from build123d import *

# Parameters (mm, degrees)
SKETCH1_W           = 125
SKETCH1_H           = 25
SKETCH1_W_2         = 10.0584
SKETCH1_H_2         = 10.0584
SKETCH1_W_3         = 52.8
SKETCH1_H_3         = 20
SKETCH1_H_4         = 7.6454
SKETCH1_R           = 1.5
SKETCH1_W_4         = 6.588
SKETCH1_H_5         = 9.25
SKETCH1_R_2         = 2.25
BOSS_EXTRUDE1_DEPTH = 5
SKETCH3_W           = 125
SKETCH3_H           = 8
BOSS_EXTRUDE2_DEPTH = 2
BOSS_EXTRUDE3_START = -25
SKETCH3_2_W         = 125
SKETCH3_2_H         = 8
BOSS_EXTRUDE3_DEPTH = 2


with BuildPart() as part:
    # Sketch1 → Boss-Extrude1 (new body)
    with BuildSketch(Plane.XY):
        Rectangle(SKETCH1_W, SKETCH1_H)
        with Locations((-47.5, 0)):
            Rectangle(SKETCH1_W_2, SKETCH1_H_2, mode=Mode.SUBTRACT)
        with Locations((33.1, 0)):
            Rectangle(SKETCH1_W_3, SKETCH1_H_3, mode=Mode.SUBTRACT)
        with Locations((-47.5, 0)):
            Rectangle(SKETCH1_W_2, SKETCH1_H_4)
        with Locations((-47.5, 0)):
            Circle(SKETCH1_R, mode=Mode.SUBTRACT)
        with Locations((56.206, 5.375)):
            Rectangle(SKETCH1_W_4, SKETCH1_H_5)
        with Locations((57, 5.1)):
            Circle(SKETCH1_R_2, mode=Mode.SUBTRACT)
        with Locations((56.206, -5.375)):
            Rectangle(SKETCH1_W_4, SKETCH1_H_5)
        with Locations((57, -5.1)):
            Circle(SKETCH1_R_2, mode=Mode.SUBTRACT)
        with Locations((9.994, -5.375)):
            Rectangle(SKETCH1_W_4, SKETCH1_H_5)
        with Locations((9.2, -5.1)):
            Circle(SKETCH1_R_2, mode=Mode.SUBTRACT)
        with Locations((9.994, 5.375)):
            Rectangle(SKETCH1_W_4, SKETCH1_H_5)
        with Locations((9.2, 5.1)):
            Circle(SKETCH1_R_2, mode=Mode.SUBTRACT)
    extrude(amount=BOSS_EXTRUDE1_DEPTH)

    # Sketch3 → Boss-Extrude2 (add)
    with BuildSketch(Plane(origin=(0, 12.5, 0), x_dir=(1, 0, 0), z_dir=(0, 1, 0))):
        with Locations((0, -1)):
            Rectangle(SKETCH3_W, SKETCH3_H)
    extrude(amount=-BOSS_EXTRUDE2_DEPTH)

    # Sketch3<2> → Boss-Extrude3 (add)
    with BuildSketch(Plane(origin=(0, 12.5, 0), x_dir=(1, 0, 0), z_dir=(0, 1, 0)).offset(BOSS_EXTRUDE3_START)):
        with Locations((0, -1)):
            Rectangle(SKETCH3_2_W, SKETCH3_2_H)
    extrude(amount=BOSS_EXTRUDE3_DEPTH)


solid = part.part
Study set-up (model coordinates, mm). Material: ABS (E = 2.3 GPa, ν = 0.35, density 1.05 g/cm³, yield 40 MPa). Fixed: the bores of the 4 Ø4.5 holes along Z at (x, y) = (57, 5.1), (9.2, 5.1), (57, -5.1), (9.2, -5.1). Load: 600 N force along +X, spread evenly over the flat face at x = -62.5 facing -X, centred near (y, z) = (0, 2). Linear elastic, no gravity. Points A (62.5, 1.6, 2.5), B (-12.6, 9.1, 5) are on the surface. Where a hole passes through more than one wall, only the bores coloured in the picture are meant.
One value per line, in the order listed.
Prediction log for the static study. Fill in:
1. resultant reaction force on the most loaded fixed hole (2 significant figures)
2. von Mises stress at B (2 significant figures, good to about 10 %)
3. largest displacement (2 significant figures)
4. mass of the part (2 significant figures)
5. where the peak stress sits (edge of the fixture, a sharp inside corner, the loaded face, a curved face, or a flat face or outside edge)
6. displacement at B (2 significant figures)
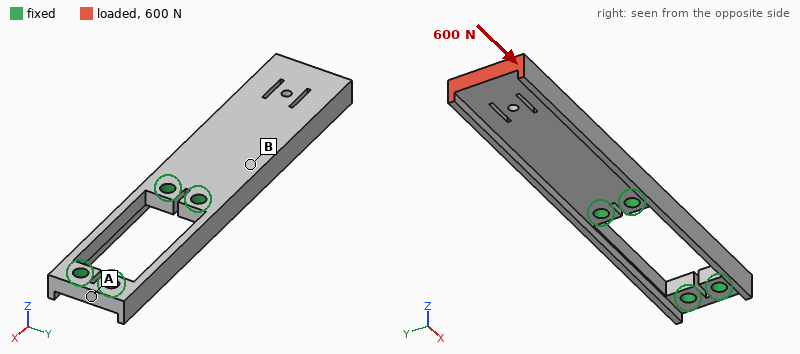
290 N
4.3 MPa
0.17 mm
13 g
a curved face
0.047 mm
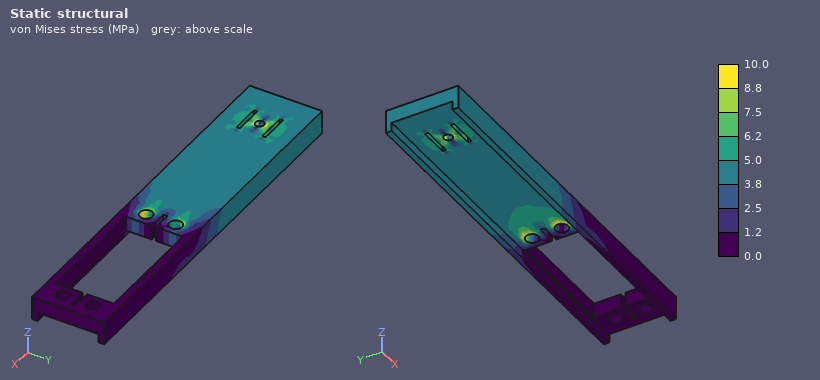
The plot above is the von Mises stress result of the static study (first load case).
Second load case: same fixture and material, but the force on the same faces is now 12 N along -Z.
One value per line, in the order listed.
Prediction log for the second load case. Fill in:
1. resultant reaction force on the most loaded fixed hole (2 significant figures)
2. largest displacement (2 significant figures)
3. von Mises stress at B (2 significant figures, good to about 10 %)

13 N
1.5 mm
3.8 MPa
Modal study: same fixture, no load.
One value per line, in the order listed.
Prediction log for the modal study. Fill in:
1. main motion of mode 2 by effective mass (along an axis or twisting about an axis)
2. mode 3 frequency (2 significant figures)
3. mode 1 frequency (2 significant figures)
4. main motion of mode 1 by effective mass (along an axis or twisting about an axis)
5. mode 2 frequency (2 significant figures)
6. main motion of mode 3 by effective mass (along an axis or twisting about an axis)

along Y
1200 Hz
290 Hz
along Z
990 Hz
twisting about X
